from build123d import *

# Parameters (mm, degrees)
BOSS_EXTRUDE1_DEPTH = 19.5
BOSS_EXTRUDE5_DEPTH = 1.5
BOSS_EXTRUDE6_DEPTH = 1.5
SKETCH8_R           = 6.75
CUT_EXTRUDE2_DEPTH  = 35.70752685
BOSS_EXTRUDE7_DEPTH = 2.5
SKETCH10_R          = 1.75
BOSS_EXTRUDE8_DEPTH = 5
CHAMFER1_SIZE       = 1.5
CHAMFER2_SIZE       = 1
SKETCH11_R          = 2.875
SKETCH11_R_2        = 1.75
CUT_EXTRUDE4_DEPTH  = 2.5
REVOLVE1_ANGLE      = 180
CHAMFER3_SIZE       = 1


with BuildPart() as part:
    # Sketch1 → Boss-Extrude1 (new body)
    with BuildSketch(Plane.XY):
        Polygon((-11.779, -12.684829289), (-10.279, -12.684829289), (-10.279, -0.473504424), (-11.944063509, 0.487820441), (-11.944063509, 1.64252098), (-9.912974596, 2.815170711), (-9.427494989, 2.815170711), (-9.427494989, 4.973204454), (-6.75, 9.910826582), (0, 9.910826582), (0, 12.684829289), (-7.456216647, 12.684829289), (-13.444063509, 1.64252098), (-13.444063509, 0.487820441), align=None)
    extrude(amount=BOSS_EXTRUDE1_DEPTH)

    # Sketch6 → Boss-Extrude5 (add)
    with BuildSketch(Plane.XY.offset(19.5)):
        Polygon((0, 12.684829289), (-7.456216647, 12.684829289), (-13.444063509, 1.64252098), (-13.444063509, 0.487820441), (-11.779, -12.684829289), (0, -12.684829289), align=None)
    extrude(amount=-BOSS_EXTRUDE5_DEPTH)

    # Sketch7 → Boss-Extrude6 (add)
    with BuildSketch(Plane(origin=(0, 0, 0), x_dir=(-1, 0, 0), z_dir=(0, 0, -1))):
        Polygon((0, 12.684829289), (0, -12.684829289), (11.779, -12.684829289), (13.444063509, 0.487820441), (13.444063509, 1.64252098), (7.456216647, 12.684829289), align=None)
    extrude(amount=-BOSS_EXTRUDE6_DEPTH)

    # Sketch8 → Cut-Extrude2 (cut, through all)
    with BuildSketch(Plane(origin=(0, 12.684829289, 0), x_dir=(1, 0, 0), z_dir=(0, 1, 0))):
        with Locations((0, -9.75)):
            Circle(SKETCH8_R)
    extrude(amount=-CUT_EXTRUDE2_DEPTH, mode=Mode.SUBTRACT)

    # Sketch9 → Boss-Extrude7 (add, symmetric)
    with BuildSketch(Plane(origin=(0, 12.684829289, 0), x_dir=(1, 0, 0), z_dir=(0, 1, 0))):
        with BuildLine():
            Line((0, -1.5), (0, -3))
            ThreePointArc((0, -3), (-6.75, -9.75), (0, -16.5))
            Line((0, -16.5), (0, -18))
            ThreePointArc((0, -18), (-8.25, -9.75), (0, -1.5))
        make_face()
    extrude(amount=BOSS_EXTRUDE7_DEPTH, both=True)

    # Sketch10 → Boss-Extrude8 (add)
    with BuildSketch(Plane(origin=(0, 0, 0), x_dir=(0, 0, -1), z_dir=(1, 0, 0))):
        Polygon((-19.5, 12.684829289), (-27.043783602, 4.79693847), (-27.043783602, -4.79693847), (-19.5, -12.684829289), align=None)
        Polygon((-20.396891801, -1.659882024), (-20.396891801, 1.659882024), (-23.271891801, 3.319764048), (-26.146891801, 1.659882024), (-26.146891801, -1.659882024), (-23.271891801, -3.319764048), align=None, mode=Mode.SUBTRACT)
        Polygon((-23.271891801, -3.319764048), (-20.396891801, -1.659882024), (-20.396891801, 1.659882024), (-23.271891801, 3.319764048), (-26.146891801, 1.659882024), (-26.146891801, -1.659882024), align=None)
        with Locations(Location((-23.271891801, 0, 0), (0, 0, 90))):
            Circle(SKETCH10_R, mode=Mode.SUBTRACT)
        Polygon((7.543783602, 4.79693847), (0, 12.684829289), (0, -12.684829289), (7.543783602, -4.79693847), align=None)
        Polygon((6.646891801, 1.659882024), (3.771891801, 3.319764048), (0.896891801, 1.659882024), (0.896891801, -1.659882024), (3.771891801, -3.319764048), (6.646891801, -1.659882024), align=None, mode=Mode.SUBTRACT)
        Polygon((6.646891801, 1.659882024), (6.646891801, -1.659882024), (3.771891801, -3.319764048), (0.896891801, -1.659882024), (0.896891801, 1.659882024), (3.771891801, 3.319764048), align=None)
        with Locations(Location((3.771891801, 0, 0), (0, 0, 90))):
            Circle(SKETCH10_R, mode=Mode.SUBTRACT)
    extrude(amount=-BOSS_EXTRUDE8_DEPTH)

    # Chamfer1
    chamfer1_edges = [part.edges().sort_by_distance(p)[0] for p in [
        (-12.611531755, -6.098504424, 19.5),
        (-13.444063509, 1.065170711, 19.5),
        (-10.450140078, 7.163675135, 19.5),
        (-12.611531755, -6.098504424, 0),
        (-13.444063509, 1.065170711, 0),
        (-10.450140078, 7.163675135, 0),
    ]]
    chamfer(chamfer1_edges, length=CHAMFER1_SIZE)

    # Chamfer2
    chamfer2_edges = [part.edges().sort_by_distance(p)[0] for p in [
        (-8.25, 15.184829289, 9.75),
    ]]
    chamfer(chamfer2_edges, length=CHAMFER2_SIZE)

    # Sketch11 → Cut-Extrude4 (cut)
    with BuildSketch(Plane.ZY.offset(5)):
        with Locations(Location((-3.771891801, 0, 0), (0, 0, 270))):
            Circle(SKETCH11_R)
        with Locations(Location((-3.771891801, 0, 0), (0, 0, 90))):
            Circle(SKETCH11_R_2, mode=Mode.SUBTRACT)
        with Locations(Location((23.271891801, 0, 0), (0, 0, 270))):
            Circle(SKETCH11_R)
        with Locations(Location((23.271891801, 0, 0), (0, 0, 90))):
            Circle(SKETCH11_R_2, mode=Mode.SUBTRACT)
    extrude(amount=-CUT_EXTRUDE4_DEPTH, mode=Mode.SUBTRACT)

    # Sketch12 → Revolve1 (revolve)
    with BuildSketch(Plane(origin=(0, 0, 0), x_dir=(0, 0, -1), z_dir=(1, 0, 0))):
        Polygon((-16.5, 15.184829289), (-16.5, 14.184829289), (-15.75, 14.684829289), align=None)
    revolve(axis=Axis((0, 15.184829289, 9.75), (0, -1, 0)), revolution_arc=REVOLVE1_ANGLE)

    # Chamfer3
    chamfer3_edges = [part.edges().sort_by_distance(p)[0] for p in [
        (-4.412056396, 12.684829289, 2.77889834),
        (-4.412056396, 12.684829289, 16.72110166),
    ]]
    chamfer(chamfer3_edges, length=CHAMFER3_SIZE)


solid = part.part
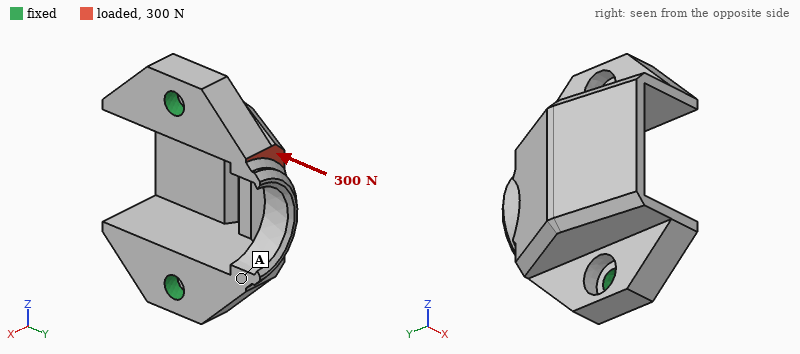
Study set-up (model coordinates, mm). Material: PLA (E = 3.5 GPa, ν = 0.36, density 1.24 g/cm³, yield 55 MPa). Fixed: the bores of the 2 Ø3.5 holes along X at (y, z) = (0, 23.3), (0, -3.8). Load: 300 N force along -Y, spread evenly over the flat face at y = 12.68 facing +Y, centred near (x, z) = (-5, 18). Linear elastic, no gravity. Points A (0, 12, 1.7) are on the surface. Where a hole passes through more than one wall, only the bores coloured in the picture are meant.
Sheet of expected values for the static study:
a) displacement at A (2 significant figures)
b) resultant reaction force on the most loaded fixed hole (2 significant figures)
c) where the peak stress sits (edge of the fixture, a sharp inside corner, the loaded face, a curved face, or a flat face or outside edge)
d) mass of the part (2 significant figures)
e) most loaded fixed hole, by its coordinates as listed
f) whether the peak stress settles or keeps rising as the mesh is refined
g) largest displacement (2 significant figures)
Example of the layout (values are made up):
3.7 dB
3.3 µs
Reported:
0.14 mm
260 N
edge of the fixture
3.8 g
(0, 23.3)
keeps rising
0.22 mm
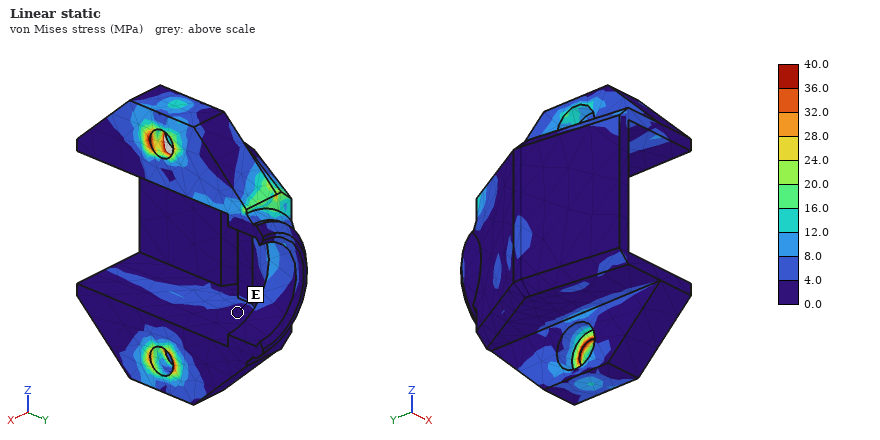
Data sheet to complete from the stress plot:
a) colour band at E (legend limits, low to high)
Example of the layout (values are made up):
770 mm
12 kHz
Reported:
0.0 to 4.0 MPa
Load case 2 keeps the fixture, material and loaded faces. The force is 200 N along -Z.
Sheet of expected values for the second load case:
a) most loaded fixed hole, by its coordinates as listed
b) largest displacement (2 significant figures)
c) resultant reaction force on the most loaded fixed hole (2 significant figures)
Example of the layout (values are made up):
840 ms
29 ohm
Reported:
(0, 23.3)
0.27 mm
140 N
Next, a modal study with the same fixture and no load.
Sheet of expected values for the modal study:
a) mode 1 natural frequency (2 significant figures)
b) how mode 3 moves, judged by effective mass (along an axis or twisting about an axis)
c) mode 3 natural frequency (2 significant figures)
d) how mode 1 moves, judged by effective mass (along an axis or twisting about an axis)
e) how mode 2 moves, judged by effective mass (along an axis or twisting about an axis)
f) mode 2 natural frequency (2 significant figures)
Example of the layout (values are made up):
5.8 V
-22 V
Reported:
2800 Hz
along Z
5800 Hz
along Y
along Z
4300 Hz
